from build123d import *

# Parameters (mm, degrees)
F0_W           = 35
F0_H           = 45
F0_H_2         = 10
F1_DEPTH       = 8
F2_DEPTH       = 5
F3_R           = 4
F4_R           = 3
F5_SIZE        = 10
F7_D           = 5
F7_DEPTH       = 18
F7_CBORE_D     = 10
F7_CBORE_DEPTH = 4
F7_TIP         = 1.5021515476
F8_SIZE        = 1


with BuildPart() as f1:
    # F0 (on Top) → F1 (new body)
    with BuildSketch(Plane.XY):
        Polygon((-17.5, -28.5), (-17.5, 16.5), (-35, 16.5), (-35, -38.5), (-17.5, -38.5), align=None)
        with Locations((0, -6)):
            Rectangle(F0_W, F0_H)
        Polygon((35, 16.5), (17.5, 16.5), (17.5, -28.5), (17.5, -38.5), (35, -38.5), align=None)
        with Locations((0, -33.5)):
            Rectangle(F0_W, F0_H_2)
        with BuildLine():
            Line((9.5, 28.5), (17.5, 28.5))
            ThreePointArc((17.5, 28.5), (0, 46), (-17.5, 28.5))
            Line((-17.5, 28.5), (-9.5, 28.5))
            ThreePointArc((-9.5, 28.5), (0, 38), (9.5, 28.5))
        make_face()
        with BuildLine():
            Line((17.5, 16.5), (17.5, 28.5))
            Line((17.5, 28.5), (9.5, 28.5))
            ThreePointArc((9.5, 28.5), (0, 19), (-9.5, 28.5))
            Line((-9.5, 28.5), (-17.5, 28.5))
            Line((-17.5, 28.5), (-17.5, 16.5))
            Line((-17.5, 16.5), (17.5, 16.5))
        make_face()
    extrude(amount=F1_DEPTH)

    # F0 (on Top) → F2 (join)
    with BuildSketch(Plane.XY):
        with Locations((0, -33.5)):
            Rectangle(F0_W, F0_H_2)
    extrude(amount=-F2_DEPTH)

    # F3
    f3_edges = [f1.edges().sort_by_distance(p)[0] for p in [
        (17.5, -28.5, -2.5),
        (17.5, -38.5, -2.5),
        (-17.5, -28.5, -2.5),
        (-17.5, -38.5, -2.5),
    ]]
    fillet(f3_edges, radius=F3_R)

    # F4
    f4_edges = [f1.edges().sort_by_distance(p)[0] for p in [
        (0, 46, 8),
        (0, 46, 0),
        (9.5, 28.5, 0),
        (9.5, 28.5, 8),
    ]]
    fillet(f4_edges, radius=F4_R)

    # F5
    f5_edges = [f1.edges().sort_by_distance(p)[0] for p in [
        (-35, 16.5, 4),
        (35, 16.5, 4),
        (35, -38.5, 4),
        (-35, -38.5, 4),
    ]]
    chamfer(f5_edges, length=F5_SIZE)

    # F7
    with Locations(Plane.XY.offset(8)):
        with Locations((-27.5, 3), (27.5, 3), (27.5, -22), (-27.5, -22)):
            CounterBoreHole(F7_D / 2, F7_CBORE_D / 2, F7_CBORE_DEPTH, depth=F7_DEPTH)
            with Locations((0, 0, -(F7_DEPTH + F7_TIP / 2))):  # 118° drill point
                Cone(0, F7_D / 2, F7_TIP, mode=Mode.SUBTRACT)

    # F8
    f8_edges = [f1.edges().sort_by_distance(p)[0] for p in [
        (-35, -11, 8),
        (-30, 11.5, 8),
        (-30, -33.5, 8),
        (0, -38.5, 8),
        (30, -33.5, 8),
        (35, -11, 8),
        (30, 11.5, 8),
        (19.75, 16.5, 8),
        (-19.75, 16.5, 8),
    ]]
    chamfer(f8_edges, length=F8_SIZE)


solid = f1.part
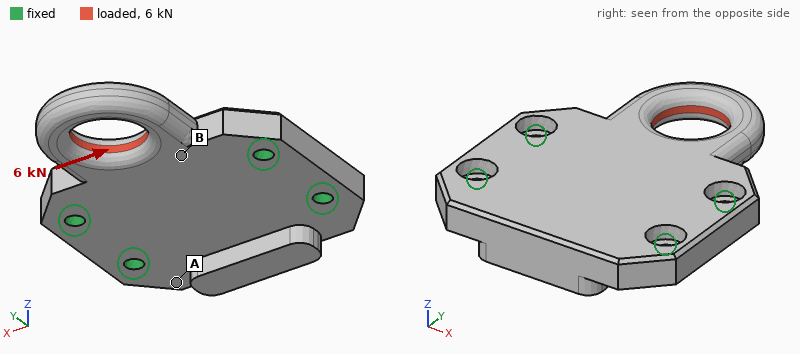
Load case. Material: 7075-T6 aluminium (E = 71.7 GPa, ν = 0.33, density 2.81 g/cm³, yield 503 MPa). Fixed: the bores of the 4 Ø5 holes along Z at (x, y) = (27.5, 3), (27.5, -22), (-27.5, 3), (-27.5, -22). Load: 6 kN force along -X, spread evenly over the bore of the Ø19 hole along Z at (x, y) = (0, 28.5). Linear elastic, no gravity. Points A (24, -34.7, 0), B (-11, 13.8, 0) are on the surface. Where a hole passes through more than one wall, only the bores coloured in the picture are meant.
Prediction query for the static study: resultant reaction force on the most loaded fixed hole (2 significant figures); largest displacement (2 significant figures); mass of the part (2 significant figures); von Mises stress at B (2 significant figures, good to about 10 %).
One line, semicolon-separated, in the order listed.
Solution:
3.4 kN; 0.10 mm; 94 g; 28 MPa
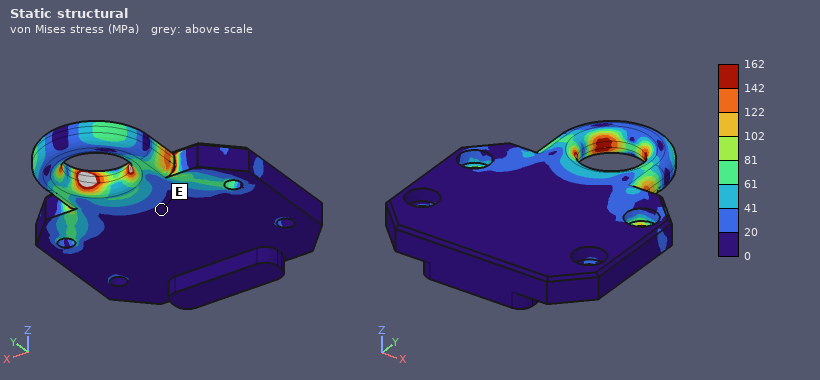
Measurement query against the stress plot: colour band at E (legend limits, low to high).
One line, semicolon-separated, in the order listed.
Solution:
0 to 20 MPa
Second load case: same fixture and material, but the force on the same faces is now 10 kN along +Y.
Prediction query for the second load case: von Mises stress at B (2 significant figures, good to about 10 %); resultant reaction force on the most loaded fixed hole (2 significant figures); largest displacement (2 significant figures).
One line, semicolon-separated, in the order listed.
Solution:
26 MPa; 2.9 kN; 54 µm
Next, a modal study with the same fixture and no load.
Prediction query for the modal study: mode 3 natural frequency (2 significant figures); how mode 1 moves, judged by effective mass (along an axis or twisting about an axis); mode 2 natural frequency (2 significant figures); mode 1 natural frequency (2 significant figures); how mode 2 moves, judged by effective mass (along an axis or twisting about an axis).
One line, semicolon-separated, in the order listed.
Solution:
9900 Hz; along Z; 7900 Hz; 3500 Hz; along Z
